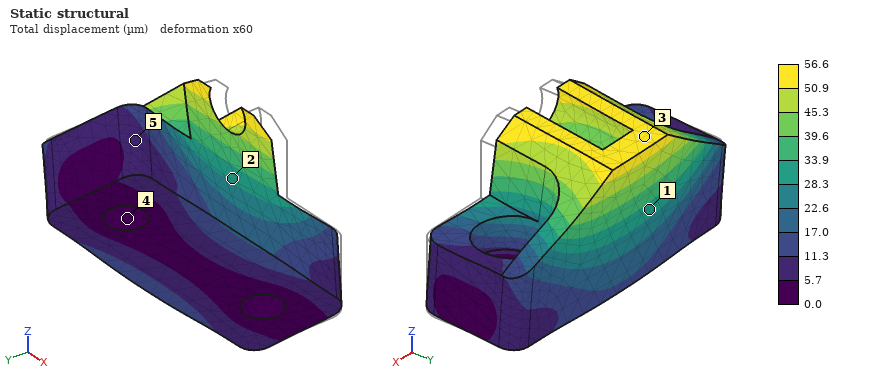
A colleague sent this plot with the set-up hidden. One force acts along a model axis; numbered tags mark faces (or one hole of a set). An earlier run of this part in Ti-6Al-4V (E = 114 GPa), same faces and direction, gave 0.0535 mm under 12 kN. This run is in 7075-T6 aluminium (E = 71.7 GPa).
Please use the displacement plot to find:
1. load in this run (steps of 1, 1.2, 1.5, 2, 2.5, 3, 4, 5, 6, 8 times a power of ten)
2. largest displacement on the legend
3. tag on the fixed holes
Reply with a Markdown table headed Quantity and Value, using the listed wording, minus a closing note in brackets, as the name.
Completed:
| Quantity | Value |
|---|---|
| load in this run | 8 kN |
| largest displacement on the legend | 56.6 µm |
| tag on the fixed holes | 4 |
